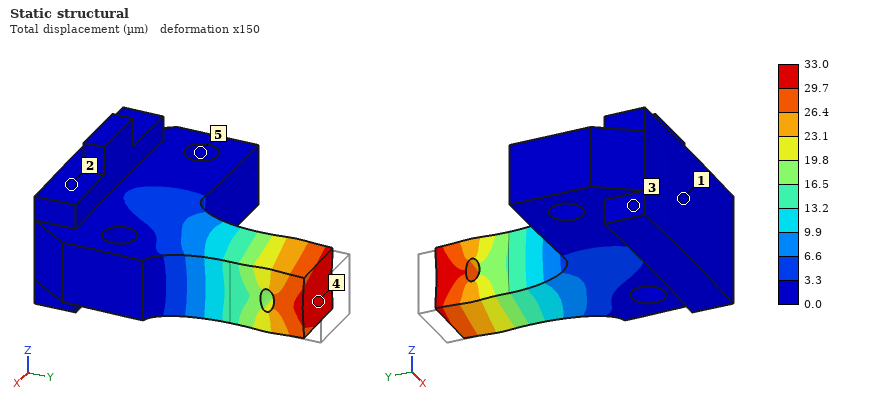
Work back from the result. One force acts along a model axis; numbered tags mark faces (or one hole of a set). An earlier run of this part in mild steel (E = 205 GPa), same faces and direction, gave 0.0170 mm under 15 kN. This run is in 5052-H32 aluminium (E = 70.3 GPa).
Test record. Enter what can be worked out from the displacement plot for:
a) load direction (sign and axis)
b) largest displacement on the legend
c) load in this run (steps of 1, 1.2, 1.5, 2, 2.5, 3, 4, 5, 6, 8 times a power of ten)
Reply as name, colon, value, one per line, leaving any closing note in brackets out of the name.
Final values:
load direction: -Y
largest displacement on the legend: 33.0 µm
load in this run: 10 kN
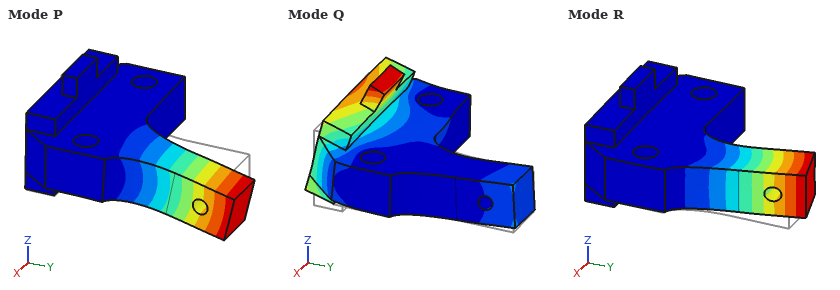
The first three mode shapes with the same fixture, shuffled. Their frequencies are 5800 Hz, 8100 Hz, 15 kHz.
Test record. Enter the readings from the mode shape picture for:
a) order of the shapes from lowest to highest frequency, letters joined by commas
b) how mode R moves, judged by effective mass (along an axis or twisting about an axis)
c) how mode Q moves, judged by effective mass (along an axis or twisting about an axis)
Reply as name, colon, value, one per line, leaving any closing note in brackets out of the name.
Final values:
order of the shapes from lowest to highest frequency, letters joined by commas: P, R, Q
how mode R moves, judged by effective mass: along X
how mode Q moves, judged by effective mass: along Z
